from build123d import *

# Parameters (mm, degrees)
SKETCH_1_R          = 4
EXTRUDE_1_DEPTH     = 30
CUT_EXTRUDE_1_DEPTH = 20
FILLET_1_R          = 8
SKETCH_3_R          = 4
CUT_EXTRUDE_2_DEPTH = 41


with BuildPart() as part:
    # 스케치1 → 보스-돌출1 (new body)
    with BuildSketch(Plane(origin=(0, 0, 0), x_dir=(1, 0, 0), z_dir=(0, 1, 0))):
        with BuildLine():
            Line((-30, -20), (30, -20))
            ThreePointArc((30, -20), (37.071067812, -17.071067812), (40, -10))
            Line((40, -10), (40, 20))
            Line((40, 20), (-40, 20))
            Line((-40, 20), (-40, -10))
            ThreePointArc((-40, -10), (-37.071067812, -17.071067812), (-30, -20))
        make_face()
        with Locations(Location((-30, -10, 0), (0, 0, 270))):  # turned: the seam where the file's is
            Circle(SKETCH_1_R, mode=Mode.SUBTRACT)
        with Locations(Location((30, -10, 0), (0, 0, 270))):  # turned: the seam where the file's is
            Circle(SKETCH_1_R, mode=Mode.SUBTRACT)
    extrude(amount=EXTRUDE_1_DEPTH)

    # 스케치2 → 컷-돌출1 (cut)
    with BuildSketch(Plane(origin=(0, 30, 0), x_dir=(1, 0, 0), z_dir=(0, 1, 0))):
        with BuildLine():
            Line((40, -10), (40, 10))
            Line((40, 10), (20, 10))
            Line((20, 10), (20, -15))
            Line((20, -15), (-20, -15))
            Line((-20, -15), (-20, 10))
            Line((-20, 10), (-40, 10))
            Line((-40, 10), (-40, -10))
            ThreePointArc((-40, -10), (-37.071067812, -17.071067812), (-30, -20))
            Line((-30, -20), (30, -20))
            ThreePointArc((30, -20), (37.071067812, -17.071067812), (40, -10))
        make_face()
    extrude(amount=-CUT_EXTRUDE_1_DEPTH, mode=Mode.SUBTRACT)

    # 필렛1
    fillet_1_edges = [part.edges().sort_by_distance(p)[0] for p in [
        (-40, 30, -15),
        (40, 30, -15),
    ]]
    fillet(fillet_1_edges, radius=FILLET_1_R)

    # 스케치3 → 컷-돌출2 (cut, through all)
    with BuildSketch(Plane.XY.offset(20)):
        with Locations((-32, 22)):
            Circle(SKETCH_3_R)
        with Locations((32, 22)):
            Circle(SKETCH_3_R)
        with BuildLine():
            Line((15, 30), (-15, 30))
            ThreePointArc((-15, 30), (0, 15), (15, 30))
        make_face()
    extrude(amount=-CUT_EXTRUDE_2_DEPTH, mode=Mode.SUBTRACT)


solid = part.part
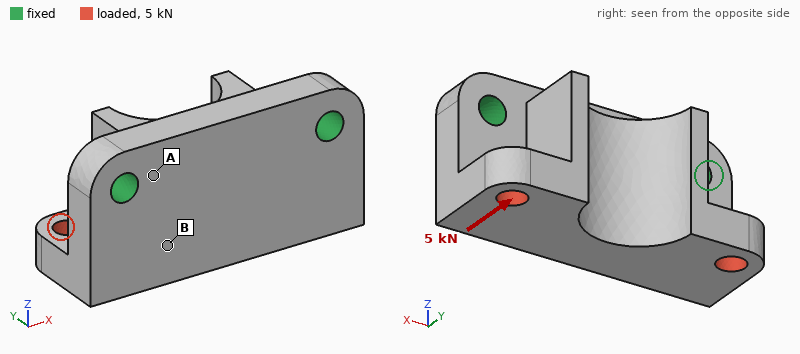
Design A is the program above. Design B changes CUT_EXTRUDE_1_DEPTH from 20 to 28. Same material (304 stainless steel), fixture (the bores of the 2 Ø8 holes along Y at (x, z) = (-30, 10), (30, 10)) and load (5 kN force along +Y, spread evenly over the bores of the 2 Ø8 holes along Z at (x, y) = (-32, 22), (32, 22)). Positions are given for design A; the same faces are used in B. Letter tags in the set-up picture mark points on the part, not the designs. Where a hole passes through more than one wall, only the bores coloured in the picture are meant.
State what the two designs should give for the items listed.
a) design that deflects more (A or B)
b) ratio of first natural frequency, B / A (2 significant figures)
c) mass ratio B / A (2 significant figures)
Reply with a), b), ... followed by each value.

a) B
b) 0.15
c) 0.81
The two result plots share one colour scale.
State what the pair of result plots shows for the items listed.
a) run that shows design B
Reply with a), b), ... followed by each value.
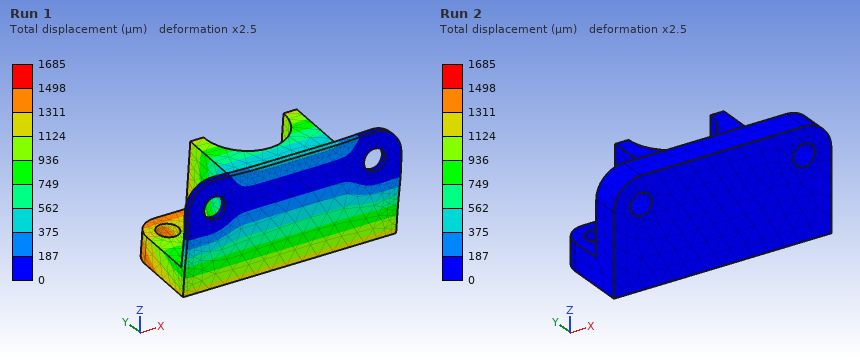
a) Run 1
